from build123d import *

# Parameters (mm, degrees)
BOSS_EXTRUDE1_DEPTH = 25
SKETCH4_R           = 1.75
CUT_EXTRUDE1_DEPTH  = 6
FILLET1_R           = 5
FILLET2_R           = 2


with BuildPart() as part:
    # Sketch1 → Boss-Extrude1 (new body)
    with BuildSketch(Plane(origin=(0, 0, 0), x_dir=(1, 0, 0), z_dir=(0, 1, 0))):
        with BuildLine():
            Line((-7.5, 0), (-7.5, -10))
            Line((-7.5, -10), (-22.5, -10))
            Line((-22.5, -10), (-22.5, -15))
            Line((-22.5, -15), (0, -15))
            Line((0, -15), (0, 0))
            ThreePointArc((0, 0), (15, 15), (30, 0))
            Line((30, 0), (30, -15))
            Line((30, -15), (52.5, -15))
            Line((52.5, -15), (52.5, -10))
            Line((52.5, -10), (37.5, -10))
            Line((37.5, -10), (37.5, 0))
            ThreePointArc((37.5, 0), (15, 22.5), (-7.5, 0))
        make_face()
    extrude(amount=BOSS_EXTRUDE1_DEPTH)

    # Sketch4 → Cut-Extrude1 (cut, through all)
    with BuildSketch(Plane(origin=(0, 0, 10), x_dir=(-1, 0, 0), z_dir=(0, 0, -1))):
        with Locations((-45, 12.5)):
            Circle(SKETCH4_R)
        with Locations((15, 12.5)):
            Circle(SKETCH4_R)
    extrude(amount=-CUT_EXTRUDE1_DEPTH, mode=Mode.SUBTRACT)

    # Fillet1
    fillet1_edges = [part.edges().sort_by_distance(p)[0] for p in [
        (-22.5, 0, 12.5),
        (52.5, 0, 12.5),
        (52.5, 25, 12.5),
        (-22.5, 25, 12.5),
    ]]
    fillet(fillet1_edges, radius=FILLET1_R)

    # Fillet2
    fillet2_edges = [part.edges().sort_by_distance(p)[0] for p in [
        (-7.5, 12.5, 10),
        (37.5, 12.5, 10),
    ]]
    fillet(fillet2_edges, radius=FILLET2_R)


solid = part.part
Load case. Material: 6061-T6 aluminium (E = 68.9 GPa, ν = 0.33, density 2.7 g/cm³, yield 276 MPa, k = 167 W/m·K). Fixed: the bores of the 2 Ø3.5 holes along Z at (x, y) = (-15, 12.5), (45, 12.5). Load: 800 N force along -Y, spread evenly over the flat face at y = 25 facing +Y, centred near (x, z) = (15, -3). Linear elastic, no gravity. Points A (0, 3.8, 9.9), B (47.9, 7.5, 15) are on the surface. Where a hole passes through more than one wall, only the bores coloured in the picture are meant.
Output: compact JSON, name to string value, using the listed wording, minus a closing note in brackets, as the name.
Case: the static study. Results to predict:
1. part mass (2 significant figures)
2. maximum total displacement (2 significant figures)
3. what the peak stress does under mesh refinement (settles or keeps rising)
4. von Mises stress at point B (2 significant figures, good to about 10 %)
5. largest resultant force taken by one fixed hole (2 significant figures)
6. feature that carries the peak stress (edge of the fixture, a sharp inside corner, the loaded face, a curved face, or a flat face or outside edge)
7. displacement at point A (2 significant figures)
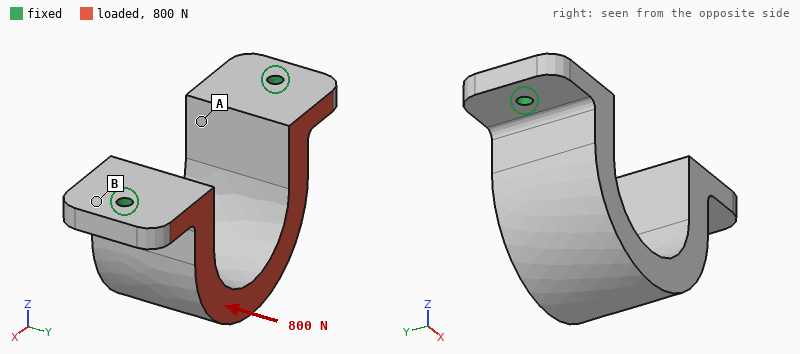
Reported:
{"part mass": "55 g", "maximum total displacement": "0.10 mm", "what the peak stress does under mesh refinement": "keeps rising", "von Mises stress at point B": "31 MPa", "largest resultant force taken by one fixed hole": "400 N", "feature that carries the peak stress": "edge of the fixture", "displacement at point A": "0.027 mm"}
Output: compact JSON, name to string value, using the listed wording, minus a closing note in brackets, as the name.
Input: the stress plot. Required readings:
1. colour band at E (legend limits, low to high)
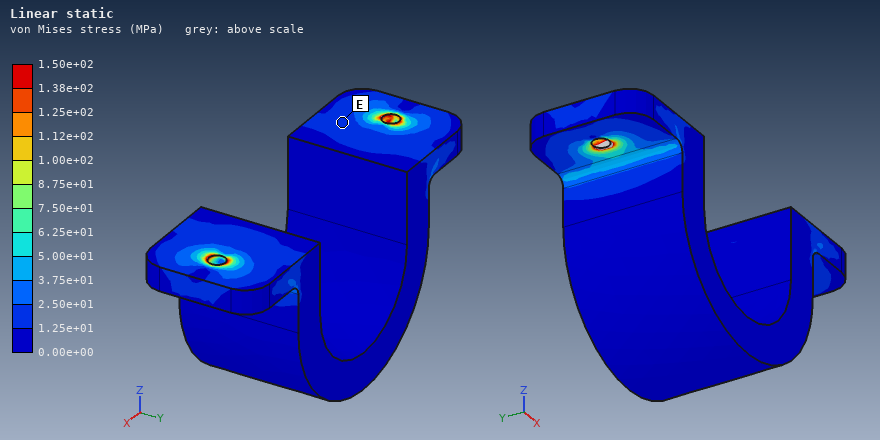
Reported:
{"colour band at E": "1.25e+01 to 2.50e+01 MPa"}
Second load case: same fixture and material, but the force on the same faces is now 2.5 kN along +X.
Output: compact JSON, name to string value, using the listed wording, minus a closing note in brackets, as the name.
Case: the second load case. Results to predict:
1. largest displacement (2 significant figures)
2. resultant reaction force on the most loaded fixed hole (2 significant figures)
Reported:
{"largest displacement": "69 µm", "resultant reaction force on the most loaded fixed hole": "1.4 kN"}
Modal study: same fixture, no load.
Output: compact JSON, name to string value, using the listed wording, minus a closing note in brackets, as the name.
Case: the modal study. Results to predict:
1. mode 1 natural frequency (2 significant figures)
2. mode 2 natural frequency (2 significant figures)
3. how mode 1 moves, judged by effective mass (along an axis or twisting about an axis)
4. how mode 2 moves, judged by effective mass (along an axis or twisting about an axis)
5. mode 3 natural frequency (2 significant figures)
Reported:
{"mode 1 natural frequency": "2300 Hz", "mode 2 natural frequency": "6000 Hz", "how mode 1 moves, judged by effective mass": "along Y", "how mode 2 moves, judged by effective mass": "along X", "mode 3 natural frequency": "8600 Hz"}
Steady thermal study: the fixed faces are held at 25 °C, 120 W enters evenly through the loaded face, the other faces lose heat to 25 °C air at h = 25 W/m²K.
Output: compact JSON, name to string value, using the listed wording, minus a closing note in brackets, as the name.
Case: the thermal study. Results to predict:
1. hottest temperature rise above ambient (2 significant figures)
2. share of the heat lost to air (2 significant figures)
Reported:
{"hottest temperature rise above ambient": "68 K", "share of the heat lost to air": "5.8 %"}
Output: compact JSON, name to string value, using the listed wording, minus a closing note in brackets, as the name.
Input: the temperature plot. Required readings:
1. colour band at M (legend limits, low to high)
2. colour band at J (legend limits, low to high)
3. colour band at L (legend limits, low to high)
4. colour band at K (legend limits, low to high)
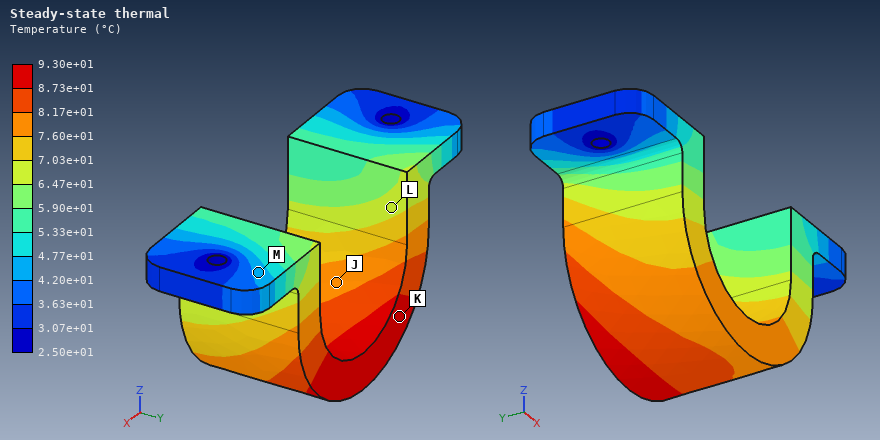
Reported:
{"colour band at M": "4.20e+01 to 4.77e+01 °C", "colour band at J": "7.60e+01 to 8.17e+01 °C", "colour band at L": "6.47e+01 to 7.03e+01 °C", "colour band at K": "8.73e+01 to 9.30e+01 °C"}
